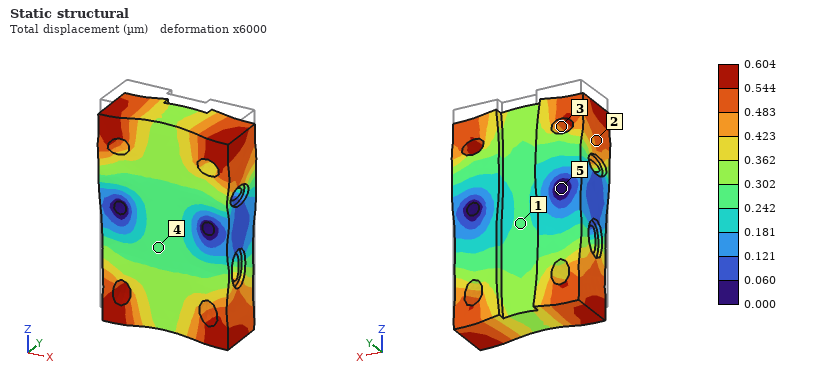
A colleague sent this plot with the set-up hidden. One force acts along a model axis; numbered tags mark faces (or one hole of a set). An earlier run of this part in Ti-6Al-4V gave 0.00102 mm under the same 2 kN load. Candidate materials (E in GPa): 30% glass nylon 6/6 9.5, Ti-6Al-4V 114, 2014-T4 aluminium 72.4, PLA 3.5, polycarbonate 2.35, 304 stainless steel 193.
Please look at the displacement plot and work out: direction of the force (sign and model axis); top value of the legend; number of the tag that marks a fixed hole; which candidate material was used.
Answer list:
-Z
0.604 µm
5
304 stainless steel
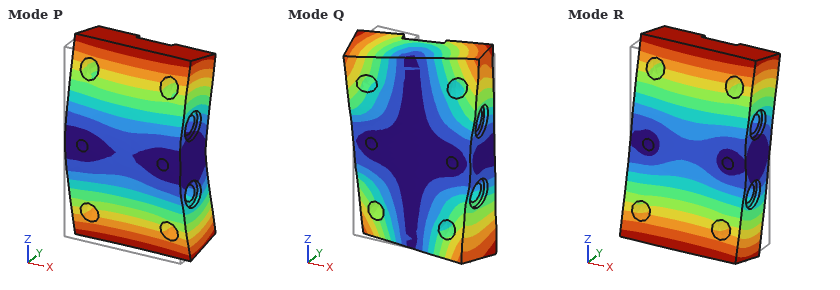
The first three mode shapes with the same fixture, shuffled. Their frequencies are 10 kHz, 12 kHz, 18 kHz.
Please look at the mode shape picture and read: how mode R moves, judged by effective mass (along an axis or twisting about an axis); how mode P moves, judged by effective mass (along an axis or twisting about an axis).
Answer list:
twisting about X
along Y
